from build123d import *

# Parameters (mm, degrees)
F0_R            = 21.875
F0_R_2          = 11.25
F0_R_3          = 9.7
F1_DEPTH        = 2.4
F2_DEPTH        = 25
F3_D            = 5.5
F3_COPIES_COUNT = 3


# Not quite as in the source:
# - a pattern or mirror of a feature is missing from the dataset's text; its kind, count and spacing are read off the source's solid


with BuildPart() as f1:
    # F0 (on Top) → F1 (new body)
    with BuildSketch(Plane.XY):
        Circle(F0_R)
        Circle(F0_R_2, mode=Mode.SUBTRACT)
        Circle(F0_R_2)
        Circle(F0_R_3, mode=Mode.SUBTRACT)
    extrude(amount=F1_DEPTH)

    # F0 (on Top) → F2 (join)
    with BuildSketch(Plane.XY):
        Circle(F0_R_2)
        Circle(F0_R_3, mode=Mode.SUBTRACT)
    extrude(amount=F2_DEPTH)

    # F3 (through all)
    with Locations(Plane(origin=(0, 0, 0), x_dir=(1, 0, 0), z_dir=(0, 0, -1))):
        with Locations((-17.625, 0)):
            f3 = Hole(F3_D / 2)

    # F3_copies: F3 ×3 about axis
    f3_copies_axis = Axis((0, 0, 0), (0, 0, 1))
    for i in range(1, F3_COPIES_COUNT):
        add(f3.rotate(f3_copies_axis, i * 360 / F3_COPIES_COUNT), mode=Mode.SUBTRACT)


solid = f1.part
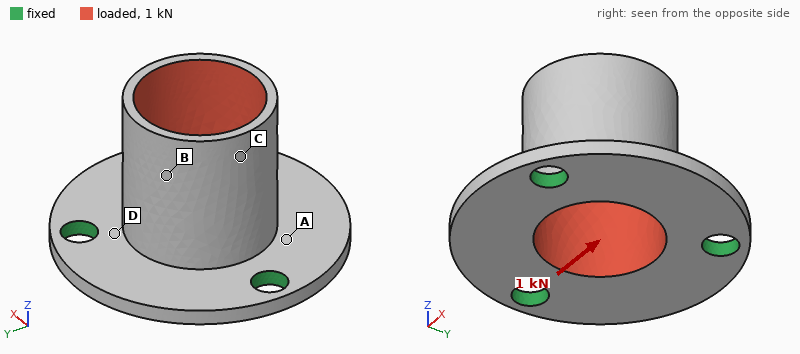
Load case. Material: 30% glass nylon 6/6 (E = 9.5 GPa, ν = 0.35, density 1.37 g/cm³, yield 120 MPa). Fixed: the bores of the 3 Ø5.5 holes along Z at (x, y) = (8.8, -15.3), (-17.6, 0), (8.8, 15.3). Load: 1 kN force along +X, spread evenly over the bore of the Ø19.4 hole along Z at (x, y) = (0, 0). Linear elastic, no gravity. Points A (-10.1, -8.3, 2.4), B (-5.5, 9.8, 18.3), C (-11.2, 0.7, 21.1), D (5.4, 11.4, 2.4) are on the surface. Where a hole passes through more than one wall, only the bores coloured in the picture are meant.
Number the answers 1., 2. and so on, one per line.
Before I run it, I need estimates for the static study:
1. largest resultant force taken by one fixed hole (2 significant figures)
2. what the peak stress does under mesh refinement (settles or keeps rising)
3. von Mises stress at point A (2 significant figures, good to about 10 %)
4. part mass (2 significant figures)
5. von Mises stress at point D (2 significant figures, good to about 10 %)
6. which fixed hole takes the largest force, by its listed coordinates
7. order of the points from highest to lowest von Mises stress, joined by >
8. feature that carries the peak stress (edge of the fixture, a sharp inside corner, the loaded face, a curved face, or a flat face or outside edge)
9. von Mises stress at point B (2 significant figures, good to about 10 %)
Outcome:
1. 600 N
2. keeps rising
3. 32 MPa
4. 6.9 g
5. 41 MPa
6. (-17.6, 0)
7. D > A > B > C
8. edge of the fixture
9. 15 MPa
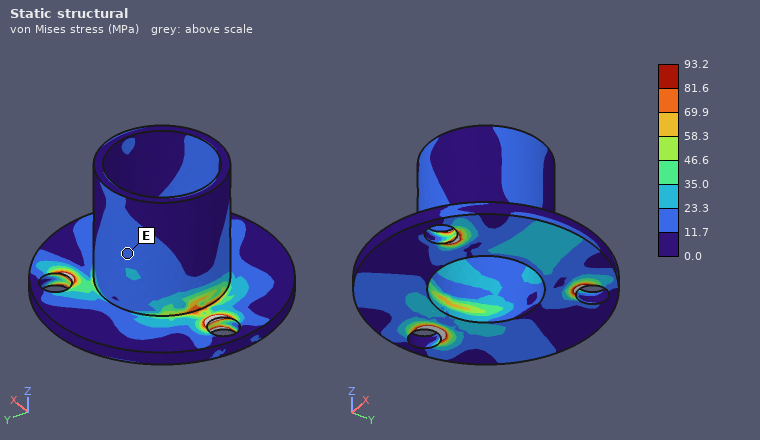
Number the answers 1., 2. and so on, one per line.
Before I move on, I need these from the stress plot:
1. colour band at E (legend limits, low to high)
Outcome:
1. 11.7 to 23.3 MPa
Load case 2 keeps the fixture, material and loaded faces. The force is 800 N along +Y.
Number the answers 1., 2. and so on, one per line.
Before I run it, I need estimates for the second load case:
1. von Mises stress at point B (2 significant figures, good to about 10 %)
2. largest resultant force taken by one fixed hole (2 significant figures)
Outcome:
1. 12 MPa
2. 430 N
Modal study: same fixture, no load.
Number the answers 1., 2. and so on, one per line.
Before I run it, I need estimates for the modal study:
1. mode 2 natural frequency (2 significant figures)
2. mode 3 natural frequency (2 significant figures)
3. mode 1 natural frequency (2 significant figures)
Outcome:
1. 4400 Hz
2. 6200 Hz
3. 4400 Hz
